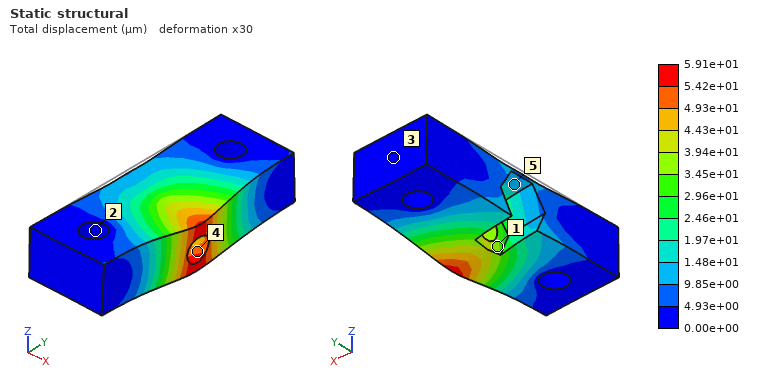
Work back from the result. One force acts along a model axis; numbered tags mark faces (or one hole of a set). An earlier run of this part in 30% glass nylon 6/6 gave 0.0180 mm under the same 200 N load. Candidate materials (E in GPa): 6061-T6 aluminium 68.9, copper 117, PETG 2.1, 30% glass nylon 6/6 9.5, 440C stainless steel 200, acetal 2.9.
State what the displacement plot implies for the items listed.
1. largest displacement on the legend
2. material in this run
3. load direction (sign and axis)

5.91e+01 µm
acetal
-Z
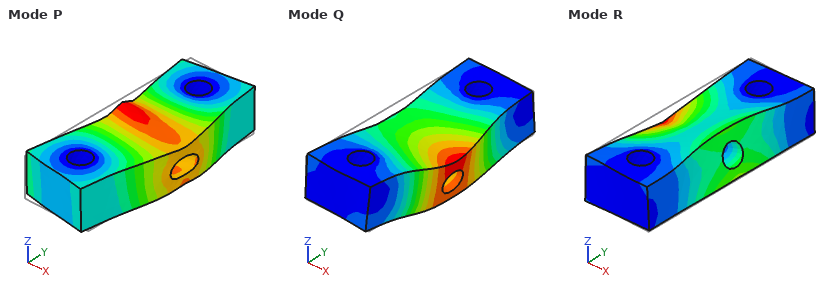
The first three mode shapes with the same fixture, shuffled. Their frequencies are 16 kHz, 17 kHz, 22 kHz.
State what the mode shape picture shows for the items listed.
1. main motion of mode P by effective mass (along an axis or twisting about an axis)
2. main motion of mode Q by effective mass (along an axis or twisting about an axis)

along X
along Z
